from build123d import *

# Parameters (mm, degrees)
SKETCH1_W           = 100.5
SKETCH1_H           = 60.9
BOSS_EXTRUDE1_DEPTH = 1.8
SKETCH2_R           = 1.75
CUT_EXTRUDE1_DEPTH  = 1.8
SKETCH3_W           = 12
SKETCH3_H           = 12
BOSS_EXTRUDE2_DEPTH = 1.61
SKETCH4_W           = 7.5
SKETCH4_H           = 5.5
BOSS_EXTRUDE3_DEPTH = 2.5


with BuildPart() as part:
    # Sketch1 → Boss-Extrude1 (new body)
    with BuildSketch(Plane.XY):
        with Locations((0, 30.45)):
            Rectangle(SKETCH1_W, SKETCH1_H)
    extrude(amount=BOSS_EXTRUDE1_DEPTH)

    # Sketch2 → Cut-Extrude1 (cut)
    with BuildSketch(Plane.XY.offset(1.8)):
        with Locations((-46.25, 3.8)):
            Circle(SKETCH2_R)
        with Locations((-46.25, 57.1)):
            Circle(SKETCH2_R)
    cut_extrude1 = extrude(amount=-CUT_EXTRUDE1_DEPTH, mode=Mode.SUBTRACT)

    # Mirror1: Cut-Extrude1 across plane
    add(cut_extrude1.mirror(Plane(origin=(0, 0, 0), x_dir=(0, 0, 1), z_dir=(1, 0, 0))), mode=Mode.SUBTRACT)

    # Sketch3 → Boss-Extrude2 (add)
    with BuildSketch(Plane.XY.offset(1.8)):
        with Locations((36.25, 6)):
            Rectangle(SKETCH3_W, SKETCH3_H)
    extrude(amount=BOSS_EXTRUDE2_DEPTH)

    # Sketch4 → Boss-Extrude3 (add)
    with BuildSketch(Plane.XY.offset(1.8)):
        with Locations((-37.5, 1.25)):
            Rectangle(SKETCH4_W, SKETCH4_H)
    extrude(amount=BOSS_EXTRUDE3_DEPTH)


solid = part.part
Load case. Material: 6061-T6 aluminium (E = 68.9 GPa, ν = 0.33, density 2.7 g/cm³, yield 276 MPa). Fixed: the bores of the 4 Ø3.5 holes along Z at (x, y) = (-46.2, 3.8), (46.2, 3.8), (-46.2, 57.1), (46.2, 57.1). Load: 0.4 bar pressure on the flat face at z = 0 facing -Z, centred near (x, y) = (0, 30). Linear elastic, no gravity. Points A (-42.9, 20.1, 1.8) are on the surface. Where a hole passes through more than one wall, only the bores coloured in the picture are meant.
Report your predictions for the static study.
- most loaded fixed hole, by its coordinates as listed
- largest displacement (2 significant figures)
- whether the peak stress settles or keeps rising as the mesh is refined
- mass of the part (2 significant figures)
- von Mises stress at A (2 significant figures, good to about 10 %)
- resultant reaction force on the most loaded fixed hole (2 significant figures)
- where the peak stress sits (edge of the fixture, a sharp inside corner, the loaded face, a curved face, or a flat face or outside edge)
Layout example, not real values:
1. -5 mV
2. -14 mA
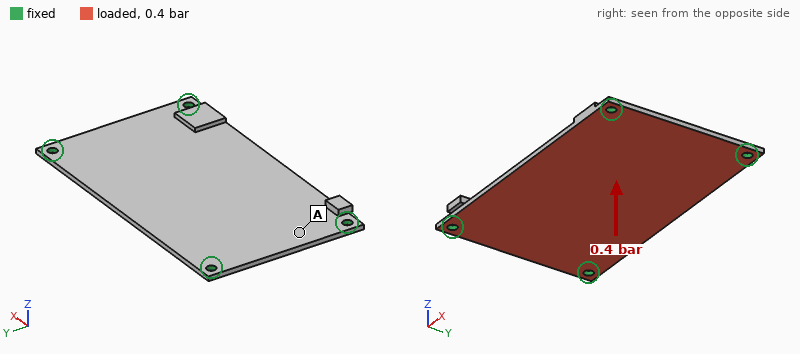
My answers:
1. (46.2, 3.8)
2. 0.31 mm
3. keeps rising
4. 30 g
5. 14 MPa
6. 71 N
7. edge of the fixture
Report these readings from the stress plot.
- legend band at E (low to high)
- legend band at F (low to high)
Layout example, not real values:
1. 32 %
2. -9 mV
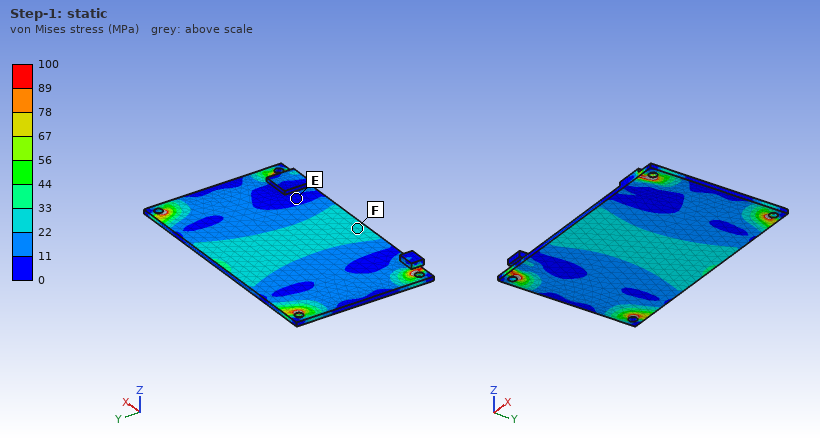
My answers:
1. 0 to 11 MPa
2. 22 to 33 MPa
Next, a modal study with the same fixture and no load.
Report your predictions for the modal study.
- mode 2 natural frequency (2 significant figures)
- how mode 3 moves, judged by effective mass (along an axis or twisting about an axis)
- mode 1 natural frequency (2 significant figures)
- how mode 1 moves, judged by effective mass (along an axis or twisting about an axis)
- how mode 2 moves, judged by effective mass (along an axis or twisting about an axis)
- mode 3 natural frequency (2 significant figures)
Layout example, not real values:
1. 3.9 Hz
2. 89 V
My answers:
1. 1600 Hz
2. twisting about Y
3. 950 Hz
4. along Z
5. twisting about X
6. 2500 Hz
